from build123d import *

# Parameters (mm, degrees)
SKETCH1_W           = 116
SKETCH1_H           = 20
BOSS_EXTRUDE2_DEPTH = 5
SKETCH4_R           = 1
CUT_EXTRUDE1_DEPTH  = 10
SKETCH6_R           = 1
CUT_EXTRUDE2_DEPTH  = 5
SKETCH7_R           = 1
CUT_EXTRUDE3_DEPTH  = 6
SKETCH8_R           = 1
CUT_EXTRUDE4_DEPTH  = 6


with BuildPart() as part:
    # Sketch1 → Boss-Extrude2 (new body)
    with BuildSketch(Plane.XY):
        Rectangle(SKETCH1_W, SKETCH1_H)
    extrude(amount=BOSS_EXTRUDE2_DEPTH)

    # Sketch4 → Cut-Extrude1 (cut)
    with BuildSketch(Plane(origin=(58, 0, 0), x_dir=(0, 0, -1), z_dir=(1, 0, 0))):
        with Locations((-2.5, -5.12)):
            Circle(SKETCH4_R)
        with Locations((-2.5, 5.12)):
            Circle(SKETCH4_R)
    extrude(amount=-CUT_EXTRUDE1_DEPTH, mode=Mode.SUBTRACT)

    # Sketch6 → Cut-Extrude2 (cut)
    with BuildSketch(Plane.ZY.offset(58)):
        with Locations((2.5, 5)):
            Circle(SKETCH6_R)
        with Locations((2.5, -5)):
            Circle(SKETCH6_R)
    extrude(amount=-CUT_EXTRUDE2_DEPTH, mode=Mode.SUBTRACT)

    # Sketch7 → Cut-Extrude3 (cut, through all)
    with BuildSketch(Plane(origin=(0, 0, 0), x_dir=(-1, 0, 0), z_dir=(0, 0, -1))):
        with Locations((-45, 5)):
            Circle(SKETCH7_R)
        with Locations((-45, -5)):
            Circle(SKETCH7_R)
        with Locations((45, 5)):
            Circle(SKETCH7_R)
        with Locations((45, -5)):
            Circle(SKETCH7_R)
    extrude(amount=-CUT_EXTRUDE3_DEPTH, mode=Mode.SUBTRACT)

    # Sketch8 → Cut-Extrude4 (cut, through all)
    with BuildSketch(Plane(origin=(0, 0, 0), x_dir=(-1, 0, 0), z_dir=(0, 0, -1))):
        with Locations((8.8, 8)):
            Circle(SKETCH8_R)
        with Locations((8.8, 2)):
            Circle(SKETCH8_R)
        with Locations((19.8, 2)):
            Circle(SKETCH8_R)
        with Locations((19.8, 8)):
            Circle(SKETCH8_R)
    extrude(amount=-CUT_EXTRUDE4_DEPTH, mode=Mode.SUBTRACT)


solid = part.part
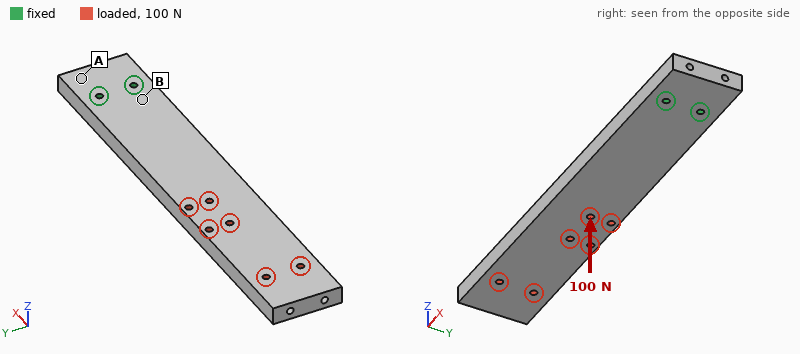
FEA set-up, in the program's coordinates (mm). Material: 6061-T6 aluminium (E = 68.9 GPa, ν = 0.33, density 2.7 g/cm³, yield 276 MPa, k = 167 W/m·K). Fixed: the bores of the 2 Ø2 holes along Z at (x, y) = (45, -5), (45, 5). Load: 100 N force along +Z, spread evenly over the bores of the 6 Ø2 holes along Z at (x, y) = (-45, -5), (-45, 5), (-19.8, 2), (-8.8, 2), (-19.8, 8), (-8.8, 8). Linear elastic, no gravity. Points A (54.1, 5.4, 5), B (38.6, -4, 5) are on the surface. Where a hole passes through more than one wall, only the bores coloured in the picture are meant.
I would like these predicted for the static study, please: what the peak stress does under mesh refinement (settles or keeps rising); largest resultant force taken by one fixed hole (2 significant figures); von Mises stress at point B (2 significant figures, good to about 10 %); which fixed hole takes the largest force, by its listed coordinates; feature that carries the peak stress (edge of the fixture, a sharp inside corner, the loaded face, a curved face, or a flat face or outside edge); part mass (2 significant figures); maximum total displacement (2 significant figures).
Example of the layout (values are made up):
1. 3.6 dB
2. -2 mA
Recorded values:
1. keeps rising
2. 74 N
3. 73 MPa
4. (45, 5)
5. edge of the fixture
6. 31 g
7. 1.4 mm
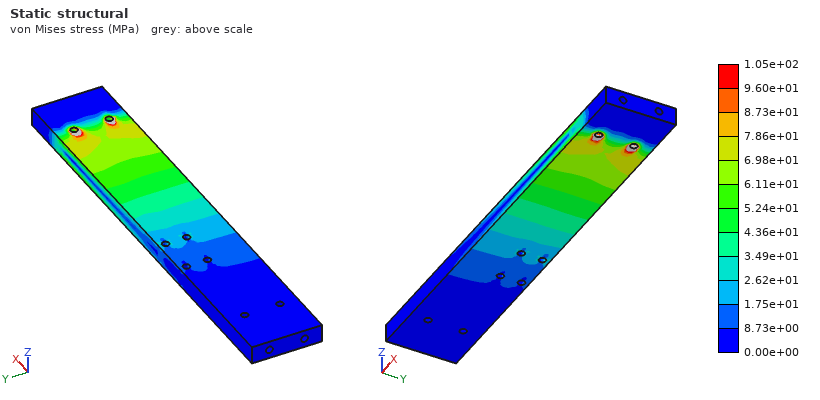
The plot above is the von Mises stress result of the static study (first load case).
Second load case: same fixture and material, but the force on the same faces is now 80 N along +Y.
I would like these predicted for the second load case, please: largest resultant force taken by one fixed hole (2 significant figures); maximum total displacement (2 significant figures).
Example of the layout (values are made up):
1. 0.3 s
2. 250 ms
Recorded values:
1. 510 N
2. 81 µm
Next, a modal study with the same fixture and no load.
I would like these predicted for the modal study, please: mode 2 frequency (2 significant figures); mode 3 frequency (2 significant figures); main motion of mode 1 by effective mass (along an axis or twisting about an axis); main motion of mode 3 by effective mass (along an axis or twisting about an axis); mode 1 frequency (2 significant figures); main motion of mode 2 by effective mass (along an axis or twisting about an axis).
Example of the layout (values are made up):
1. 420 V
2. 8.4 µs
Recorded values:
1. 1400 Hz
2. 2300 Hz
3. along Z
4. along Z
5. 380 Hz
6. along Y
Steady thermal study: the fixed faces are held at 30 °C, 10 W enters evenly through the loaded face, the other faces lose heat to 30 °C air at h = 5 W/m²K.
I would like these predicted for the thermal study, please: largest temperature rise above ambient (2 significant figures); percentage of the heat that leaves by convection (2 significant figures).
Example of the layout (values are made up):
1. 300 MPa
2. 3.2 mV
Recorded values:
1. 40 K
2. 6.9 %
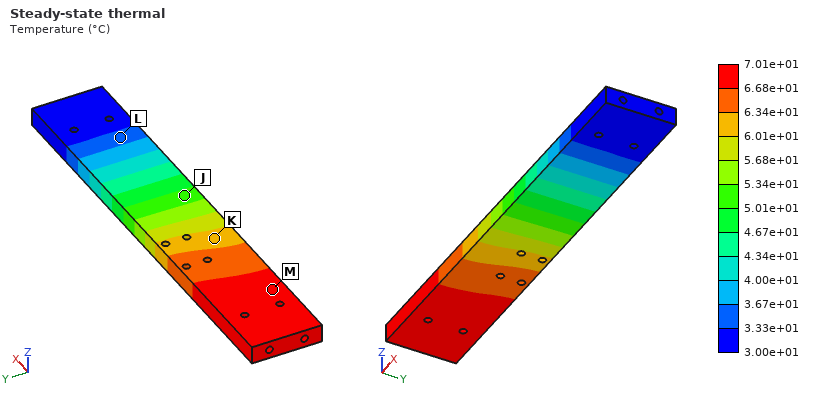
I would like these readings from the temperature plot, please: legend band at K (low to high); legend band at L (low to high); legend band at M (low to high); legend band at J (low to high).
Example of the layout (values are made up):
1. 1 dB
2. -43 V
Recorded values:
1. 6.01e+01 to 6.34e+01 °C
2. 3.33e+01 to 3.67e+01 °C
3. 6.68e+01 to 7.01e+01 °C
4. 5.01e+01 to 5.34e+01 °C
